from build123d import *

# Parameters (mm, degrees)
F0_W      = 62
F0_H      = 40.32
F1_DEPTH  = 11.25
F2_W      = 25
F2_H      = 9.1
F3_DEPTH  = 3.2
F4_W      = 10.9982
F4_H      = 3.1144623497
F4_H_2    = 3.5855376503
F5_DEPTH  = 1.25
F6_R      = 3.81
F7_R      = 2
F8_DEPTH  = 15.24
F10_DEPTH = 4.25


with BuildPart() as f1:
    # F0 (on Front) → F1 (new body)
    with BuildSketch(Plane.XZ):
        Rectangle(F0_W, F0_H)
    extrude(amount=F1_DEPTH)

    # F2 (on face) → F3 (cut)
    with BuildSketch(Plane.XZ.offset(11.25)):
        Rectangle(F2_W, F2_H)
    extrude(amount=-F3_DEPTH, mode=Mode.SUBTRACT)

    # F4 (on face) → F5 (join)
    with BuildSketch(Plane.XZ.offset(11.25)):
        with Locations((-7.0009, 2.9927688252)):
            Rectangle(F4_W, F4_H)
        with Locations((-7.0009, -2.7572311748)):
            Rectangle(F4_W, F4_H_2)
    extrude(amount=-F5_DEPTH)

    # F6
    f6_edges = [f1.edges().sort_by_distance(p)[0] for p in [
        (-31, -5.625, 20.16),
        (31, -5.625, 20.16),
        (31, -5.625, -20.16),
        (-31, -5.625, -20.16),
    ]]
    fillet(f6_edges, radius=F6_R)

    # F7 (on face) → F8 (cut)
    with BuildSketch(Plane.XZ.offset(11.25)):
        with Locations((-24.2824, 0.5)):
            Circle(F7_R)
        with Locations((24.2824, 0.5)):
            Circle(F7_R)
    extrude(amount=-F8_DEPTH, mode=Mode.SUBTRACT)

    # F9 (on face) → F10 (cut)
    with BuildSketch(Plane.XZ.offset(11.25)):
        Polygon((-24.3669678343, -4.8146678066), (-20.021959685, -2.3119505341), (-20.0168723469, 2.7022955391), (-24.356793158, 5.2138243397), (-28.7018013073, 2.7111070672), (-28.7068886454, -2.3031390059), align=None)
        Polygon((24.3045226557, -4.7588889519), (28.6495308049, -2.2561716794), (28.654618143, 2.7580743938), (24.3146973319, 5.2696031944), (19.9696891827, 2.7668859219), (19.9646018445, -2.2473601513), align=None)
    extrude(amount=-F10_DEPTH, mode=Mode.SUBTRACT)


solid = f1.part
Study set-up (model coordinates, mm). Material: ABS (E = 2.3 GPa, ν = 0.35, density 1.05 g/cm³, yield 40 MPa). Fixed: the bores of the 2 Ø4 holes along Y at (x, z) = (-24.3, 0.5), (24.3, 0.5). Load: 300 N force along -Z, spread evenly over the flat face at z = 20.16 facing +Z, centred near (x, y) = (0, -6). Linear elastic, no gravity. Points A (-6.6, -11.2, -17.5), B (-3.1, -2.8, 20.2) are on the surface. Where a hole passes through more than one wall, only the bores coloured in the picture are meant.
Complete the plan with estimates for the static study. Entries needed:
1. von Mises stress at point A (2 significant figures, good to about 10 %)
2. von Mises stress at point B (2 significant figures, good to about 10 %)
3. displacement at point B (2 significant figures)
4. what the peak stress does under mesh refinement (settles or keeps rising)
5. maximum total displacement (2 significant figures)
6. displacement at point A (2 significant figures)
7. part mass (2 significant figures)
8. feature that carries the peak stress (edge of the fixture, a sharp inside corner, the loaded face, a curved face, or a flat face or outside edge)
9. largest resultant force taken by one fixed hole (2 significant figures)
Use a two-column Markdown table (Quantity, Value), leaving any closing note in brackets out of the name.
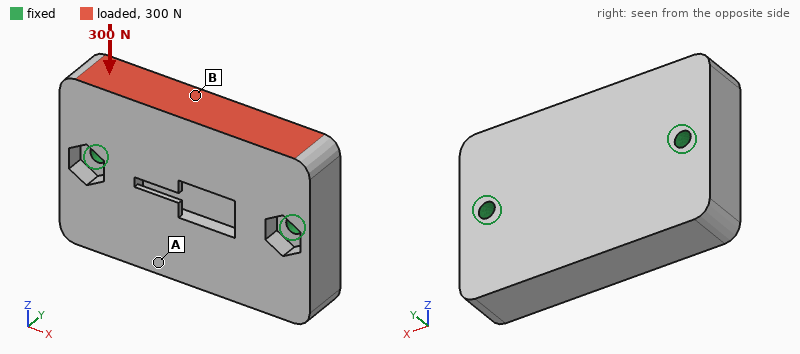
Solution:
| Quantity | Value |
|---|---|
| von Mises stress at point A | 0.34 MPa |
| von Mises stress at point B | 0.64 MPa |
| displacement at point B | 23 µm |
| what the peak stress does under mesh refinement | keeps rising |
| maximum total displacement | 30 µm |
| displacement at point A | 21 µm |
| part mass | 28 g |
| feature that carries the peak stress | edge of the fixture |
| largest resultant force taken by one fixed hole | 150 N |
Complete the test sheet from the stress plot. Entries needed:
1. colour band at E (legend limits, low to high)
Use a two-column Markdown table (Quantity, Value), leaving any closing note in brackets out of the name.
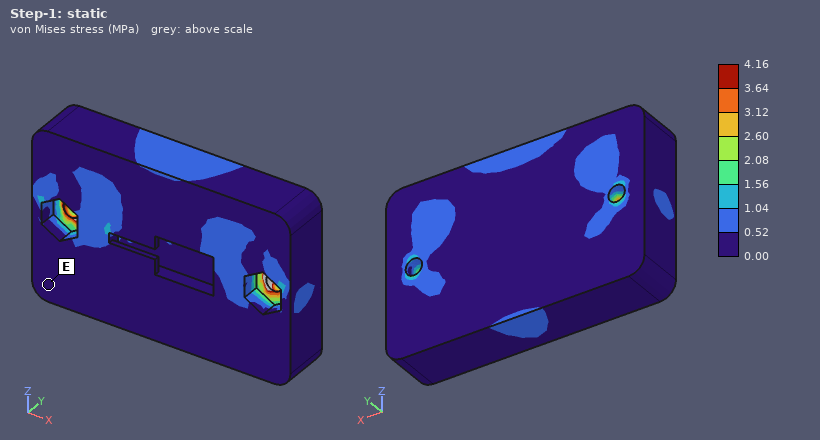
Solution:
| Quantity | Value |
|---|---|
| colour band at E | 0.00 to 0.52 MPa |
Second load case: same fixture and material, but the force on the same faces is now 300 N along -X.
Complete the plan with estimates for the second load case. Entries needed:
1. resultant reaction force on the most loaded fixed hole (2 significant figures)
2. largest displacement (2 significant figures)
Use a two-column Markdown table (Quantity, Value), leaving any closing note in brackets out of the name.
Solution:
| Quantity | Value |
|---|---|
| resultant reaction force on the most loaded fixed hole | 190 N |
| largest displacement | 22 µm |
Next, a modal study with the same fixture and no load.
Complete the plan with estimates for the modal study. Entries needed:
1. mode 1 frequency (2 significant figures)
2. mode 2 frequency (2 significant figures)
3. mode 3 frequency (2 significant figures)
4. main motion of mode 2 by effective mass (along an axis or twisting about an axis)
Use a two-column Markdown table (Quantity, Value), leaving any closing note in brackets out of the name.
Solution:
| Quantity | Value |
|---|---|
| mode 1 frequency | 2000 Hz |
| mode 2 frequency | 3100 Hz |
| mode 3 frequency | 4300 Hz |
| main motion of mode 2 by effective mass | along Y |
